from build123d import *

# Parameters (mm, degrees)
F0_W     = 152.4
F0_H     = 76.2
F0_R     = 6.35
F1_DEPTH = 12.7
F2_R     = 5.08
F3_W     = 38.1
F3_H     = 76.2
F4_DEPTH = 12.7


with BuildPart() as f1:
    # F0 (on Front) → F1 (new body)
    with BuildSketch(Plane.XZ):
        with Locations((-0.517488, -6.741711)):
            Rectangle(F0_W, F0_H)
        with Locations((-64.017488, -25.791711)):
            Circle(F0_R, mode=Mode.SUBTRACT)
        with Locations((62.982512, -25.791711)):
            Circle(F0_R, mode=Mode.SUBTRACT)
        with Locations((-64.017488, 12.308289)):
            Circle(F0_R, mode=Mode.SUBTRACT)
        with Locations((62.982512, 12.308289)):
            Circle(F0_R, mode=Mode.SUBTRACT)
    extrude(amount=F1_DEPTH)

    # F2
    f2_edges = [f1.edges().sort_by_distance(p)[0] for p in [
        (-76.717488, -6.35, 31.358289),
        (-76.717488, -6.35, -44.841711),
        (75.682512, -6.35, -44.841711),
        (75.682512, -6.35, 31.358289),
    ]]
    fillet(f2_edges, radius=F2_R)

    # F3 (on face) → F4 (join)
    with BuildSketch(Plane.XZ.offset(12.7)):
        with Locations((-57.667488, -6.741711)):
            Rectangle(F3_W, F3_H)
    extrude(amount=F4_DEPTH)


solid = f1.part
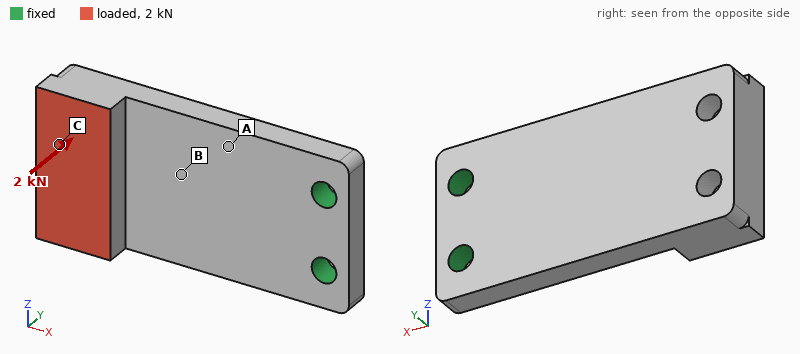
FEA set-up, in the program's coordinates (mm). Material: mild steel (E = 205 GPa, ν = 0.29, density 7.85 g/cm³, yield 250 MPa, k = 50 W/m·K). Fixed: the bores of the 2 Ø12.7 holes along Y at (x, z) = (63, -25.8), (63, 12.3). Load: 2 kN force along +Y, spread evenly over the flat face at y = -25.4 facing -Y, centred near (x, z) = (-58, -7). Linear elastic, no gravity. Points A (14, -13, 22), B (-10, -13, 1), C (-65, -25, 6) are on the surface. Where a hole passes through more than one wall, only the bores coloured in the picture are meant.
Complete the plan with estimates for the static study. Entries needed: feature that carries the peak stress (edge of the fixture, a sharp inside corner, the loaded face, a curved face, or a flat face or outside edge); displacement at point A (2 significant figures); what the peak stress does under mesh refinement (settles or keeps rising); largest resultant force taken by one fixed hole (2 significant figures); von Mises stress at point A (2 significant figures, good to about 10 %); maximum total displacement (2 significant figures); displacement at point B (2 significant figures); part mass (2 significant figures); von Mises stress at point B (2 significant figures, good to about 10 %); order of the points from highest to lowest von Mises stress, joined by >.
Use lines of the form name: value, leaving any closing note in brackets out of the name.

feature that carries the peak stress: edge of the fixture
displacement at point A: 0.083 mm
what the peak stress does under mesh refinement: keeps rising
largest resultant force taken by one fixed hole: 1.0 kN
von Mises stress at point A: 70 MPa
maximum total displacement: 0.51 mm
displacement at point B: 0.18 mm
part mass: 1.4 kg
von Mises stress at point B: 44 MPa
order of the points from highest to lowest von Mises stress, joined by >: A > B > C
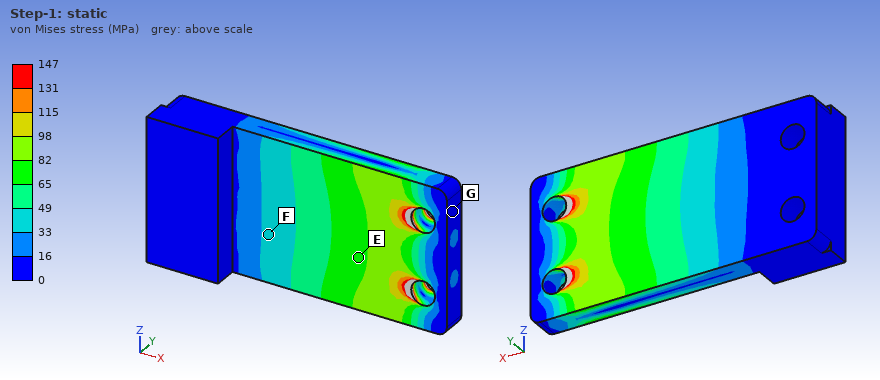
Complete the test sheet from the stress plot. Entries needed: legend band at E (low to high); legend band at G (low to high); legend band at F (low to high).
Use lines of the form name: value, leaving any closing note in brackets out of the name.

legend band at E: 65 to 82 MPa
legend band at G: 0 to 16 MPa
legend band at F: 33 to 49 MPa
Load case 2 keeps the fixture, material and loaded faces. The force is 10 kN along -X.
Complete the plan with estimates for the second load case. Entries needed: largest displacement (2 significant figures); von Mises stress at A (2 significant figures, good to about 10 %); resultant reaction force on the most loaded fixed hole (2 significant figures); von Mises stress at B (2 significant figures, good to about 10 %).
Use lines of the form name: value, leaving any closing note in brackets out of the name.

largest displacement: 0.64 mm
von Mises stress at A: 100 MPa
resultant reaction force on the most loaded fixed hole: 5.0 kN
von Mises stress at B: 98 MPa
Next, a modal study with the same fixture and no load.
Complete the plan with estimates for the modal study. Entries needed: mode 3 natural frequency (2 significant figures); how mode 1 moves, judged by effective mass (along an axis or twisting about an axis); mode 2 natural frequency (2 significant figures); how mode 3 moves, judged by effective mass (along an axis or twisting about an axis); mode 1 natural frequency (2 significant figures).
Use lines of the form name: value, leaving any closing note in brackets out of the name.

mode 3 natural frequency: 2100 Hz
how mode 1 moves, judged by effective mass: along Y
mode 2 natural frequency: 1600 Hz
how mode 3 moves, judged by effective mass: along Z
mode 1 natural frequency: 430 Hz
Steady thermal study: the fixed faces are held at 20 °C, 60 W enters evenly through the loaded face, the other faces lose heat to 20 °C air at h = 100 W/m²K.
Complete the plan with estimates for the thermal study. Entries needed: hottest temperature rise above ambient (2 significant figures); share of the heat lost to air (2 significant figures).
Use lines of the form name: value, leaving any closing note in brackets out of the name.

hottest temperature rise above ambient: 42 K
share of the heat lost to air: 86 %
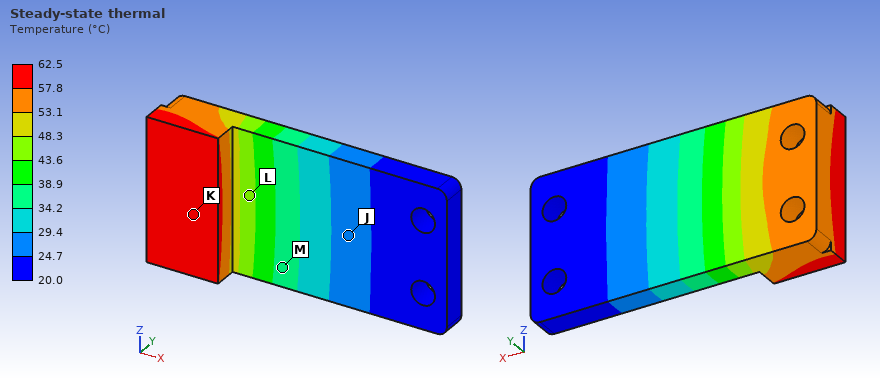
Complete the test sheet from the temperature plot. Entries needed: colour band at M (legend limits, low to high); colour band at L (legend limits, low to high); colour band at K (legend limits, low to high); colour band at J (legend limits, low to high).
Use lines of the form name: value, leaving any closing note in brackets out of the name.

colour band at M: 34.2 to 38.9 °C
colour band at L: 43.6 to 48.3 °C
colour band at K: 57.8 to 62.5 °C
colour band at J: 24.7 to 29.4 °C
